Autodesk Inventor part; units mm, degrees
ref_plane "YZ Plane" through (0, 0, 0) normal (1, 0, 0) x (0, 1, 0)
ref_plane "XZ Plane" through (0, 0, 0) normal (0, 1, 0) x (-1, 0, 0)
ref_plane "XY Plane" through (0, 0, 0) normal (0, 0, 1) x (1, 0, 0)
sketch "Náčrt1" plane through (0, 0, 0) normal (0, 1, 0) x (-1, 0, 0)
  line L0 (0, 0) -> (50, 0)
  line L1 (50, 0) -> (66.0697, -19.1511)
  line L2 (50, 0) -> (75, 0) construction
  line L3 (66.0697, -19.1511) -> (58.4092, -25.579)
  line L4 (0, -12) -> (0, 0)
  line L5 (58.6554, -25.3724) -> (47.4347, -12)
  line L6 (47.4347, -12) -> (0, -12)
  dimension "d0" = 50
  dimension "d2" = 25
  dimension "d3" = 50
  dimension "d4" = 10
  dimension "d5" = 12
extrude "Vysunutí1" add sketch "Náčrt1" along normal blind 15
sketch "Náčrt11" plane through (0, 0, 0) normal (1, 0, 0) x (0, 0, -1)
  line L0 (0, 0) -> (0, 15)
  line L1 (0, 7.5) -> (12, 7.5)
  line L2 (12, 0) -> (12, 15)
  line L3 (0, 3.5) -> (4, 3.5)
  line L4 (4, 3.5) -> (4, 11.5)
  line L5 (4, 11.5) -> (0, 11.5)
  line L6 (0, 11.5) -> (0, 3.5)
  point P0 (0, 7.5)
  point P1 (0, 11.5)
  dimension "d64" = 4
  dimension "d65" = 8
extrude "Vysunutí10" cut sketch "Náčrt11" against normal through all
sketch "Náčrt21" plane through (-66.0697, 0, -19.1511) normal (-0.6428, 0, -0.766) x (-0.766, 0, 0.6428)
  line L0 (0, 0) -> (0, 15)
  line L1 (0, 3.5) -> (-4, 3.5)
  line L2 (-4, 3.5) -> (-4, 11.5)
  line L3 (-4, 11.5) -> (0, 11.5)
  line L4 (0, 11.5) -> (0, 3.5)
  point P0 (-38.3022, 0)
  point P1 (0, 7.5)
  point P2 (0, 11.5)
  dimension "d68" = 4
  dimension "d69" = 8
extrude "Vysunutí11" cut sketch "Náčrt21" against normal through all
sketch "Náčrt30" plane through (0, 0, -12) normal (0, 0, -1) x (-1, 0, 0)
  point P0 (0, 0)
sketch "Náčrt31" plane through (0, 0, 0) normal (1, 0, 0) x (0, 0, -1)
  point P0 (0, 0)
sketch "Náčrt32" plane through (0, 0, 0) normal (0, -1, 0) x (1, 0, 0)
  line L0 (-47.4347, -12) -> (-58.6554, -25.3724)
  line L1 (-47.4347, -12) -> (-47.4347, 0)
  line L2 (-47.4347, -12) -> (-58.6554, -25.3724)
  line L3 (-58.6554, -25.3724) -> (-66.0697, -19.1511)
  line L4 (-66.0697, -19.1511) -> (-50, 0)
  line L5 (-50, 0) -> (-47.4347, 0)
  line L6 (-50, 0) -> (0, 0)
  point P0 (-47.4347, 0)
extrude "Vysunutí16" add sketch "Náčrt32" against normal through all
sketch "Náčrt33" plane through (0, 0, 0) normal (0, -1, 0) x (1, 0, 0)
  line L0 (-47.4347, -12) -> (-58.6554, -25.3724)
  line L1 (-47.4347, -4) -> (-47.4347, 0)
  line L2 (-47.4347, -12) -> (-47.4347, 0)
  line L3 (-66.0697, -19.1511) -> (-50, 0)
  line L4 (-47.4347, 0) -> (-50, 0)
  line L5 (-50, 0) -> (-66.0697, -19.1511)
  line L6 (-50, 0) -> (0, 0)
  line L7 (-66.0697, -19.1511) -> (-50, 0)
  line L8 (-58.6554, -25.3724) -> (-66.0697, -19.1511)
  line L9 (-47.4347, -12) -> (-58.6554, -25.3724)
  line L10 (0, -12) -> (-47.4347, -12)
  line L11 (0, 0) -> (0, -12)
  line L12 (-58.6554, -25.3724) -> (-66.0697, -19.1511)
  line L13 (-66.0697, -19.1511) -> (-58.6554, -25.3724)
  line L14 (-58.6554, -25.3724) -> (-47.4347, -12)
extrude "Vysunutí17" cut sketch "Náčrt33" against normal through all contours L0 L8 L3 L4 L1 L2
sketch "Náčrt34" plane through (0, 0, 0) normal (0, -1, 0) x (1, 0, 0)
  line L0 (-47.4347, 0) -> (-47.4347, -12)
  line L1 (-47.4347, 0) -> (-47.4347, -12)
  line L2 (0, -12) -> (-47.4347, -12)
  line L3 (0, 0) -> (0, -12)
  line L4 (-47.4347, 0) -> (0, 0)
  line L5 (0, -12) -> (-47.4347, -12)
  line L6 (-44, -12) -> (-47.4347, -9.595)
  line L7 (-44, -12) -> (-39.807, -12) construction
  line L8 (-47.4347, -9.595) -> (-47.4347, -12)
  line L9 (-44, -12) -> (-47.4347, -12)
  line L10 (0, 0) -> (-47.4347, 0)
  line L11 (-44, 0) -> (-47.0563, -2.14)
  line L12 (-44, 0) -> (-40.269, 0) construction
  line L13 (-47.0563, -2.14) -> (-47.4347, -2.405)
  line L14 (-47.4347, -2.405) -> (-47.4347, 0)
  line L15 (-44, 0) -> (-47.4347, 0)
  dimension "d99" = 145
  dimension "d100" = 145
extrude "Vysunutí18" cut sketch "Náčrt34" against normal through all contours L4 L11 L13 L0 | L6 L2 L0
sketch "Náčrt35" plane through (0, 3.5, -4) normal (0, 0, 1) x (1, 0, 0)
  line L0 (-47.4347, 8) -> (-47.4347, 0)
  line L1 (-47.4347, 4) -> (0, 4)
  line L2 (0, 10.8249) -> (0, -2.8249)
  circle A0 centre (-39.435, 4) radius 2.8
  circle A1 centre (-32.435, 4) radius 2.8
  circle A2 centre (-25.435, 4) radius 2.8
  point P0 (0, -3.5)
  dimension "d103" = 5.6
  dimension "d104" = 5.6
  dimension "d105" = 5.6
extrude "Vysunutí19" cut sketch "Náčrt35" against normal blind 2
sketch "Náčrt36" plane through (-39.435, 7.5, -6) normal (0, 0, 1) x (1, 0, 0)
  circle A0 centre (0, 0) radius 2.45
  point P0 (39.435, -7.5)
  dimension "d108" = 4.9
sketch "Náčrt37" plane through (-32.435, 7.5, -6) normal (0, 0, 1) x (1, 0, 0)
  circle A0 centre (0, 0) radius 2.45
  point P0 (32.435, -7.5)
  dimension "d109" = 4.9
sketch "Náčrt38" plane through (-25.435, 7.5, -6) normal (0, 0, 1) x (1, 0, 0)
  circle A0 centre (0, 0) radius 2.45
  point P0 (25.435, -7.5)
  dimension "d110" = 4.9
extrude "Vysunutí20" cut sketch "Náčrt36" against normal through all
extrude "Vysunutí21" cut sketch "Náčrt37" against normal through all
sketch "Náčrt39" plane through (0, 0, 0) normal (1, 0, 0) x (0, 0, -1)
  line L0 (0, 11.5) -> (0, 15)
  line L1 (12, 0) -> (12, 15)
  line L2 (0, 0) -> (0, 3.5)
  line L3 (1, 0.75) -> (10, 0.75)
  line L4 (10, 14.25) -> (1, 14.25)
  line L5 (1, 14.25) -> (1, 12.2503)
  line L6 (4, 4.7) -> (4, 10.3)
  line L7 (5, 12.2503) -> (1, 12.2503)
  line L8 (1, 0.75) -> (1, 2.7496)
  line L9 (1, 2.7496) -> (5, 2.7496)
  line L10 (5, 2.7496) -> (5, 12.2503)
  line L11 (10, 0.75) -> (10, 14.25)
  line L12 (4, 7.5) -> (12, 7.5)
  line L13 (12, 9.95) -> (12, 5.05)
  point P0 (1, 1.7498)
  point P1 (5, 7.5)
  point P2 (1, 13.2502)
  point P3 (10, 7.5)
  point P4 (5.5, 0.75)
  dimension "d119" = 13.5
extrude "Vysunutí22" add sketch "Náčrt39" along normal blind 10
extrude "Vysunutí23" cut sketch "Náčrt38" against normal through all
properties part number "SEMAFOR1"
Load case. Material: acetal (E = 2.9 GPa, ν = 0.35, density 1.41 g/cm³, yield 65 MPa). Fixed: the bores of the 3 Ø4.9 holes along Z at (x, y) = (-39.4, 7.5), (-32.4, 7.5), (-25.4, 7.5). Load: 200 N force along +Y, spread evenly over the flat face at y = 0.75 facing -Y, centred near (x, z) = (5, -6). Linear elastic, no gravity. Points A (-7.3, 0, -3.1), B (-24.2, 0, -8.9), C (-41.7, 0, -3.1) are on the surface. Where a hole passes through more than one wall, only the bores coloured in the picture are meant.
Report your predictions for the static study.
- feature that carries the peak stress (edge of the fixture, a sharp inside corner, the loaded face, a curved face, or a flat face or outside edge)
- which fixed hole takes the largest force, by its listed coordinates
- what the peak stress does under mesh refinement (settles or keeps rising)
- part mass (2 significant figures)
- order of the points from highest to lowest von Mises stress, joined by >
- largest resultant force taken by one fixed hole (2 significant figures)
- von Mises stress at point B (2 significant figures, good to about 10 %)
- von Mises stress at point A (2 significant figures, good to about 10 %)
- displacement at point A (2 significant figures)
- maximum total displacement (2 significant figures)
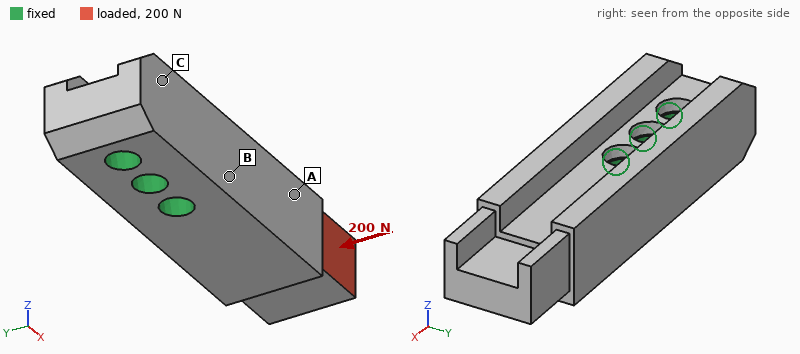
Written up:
edge of the fixture
(-25.4, 7.5)
keeps rising
10 g
B > A > C
480 N
14 MPa
6.6 MPa
0.24 mm
0.66 mm
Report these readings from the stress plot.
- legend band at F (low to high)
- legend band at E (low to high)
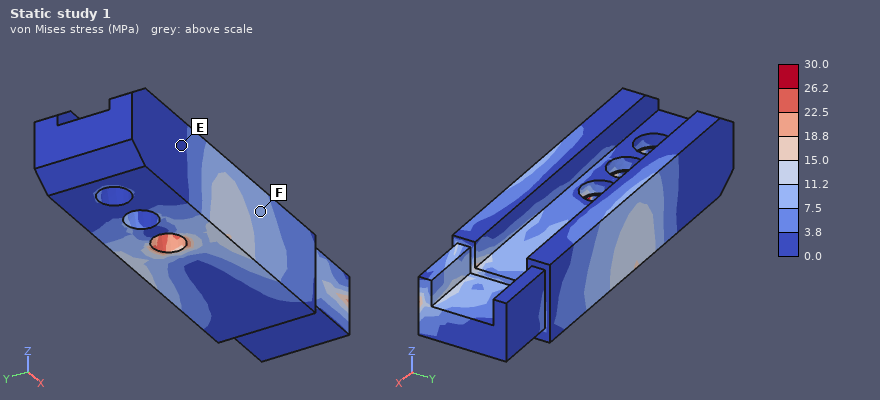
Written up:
7.5 to 11.2 MPa
0.0 to 3.8 MPa
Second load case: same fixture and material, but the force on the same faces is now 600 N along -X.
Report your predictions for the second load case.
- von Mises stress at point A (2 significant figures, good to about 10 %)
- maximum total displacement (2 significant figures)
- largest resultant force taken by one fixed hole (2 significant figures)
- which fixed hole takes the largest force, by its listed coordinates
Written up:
16 MPa
0.56 mm
450 N
(-25.4, 7.5)
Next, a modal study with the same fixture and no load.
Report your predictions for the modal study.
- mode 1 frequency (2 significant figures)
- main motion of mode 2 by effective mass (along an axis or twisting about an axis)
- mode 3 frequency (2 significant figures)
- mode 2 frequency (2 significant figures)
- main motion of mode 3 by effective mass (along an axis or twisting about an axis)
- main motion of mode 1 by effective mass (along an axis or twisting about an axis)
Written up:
2000 Hz
along Y
4500 Hz
2400 Hz
twisting about X
along Z
